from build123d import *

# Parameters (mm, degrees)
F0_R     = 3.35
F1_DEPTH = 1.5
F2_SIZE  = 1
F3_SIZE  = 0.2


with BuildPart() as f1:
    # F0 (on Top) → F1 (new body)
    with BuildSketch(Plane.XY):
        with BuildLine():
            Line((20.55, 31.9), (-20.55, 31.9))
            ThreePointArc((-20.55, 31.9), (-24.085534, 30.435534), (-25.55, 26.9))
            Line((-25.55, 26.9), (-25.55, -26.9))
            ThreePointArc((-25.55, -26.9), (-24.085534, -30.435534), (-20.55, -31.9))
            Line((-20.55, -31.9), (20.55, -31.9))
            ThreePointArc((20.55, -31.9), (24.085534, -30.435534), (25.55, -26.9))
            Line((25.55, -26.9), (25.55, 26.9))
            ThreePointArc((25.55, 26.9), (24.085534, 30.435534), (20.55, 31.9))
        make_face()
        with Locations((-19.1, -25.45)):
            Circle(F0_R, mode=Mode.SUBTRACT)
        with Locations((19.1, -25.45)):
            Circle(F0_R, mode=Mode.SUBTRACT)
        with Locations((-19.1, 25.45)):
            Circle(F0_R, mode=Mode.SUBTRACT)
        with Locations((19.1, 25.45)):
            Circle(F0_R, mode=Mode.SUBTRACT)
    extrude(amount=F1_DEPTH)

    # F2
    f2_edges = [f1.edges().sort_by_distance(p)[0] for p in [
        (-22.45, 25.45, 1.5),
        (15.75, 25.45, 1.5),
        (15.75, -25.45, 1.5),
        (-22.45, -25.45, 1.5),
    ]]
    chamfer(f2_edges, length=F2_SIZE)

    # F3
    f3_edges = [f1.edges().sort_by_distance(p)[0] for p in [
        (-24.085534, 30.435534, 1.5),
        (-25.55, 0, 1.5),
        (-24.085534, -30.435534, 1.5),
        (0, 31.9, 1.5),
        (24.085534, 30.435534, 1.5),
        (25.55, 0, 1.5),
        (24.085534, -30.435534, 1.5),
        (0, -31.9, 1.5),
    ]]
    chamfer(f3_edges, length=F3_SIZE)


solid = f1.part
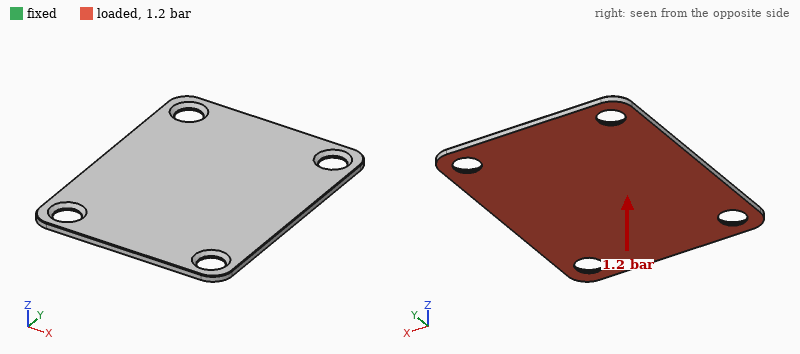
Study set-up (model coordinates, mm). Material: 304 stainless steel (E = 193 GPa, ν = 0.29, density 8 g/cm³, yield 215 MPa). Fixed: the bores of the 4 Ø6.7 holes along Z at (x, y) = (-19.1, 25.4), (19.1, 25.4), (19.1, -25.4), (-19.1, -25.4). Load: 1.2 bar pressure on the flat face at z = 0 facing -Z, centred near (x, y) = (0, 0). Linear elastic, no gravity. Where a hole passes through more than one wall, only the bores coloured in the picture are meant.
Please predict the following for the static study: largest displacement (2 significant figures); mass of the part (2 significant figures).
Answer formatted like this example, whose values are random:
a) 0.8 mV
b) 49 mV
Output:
a) 53 µm
b) 37 g
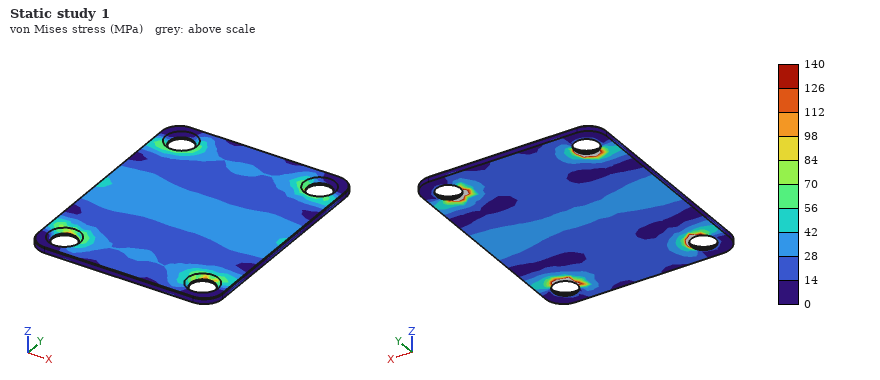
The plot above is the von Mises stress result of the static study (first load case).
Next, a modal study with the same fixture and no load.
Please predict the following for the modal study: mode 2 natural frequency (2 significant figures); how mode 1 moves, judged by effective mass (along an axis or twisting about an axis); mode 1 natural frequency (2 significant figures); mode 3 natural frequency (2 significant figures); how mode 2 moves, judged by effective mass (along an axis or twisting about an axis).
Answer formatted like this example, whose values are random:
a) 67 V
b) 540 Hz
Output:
a) 3700 Hz
b) along Z
c) 2600 Hz
d) 5000 Hz
e) twisting about Y
